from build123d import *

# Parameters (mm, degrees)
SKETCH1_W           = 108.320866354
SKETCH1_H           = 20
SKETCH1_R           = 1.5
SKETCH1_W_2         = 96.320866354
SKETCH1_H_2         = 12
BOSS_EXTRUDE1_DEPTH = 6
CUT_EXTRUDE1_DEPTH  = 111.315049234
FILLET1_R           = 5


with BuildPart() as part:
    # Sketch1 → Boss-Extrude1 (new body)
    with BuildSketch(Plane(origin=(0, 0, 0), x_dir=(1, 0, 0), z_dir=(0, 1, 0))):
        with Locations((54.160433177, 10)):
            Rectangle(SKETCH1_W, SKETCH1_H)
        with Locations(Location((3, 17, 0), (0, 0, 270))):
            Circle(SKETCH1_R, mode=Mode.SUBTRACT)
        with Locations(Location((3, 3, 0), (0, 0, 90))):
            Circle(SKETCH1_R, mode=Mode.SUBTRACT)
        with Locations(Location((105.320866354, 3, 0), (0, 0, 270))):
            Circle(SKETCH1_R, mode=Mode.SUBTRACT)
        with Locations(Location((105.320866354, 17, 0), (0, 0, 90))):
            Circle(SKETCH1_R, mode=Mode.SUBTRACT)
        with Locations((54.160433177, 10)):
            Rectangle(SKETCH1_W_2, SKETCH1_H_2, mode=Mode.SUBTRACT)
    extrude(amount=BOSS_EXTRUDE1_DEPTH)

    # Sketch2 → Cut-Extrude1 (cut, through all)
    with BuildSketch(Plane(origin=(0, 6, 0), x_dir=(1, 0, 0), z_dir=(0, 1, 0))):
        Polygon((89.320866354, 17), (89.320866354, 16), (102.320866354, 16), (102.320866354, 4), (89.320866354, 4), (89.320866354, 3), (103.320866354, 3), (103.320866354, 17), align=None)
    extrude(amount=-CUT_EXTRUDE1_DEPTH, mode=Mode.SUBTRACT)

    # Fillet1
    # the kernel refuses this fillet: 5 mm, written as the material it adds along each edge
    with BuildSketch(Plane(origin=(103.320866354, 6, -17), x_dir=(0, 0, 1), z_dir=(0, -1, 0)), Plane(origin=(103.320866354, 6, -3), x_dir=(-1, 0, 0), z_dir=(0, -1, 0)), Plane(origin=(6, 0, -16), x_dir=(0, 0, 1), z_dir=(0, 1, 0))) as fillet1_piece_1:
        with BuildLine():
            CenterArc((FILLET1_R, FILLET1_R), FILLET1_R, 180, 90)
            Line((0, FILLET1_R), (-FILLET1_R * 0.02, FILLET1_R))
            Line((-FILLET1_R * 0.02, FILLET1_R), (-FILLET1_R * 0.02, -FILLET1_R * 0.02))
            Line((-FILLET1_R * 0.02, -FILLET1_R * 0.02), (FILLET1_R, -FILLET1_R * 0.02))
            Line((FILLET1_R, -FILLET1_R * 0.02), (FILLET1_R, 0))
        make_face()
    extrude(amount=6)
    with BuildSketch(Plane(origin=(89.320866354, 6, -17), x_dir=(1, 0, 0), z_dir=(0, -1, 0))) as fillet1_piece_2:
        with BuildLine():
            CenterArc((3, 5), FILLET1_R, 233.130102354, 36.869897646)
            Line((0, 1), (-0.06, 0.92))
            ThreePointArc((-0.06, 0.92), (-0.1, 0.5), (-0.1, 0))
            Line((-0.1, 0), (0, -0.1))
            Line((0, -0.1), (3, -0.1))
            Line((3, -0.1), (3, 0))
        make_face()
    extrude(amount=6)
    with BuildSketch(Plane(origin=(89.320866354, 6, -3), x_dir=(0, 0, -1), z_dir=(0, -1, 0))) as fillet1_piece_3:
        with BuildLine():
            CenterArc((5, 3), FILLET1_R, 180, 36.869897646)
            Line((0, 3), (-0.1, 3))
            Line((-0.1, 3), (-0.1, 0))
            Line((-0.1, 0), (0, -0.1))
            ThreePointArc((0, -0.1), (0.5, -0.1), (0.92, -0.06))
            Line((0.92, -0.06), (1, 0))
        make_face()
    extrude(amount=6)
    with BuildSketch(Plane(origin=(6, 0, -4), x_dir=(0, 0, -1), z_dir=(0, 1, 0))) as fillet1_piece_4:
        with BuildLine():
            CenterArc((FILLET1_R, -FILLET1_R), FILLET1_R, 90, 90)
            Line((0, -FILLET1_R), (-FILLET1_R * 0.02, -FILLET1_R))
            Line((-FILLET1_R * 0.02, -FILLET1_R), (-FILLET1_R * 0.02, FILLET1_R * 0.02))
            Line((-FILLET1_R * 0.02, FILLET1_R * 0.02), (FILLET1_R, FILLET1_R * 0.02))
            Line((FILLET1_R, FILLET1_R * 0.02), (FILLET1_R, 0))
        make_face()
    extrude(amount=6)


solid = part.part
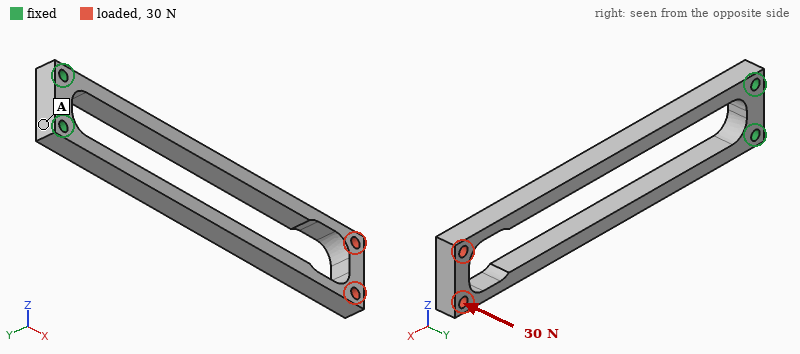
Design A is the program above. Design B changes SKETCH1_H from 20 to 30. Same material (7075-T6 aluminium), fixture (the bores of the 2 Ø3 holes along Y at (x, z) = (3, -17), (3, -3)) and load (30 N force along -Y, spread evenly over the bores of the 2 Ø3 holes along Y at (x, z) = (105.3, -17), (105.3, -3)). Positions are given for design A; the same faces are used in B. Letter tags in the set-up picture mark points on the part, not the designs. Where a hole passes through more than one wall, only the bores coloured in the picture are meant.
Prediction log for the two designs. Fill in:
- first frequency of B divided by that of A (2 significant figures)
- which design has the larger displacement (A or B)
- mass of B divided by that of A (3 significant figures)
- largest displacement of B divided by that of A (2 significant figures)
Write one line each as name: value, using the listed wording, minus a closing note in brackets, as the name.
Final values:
first frequency of B divided by that of A: 1.0
which design has the larger displacement: A
mass of B divided by that of A: 2.12
largest displacement of B divided by that of A: 0.47
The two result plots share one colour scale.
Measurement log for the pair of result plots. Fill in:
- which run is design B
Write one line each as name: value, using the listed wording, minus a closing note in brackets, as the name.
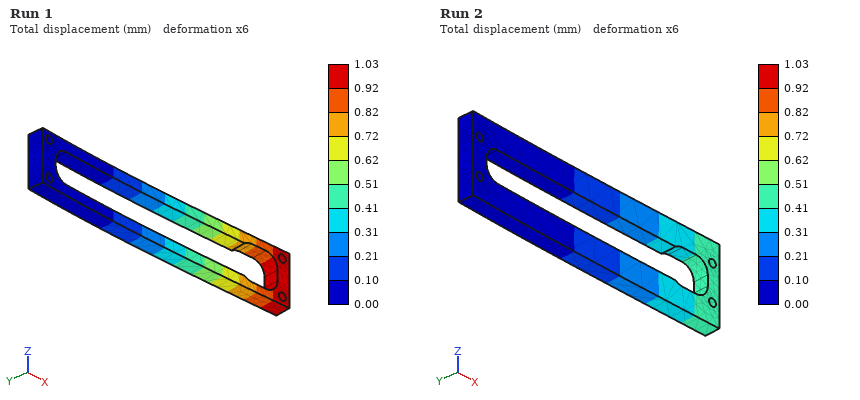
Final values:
which run is design B: Run 2
